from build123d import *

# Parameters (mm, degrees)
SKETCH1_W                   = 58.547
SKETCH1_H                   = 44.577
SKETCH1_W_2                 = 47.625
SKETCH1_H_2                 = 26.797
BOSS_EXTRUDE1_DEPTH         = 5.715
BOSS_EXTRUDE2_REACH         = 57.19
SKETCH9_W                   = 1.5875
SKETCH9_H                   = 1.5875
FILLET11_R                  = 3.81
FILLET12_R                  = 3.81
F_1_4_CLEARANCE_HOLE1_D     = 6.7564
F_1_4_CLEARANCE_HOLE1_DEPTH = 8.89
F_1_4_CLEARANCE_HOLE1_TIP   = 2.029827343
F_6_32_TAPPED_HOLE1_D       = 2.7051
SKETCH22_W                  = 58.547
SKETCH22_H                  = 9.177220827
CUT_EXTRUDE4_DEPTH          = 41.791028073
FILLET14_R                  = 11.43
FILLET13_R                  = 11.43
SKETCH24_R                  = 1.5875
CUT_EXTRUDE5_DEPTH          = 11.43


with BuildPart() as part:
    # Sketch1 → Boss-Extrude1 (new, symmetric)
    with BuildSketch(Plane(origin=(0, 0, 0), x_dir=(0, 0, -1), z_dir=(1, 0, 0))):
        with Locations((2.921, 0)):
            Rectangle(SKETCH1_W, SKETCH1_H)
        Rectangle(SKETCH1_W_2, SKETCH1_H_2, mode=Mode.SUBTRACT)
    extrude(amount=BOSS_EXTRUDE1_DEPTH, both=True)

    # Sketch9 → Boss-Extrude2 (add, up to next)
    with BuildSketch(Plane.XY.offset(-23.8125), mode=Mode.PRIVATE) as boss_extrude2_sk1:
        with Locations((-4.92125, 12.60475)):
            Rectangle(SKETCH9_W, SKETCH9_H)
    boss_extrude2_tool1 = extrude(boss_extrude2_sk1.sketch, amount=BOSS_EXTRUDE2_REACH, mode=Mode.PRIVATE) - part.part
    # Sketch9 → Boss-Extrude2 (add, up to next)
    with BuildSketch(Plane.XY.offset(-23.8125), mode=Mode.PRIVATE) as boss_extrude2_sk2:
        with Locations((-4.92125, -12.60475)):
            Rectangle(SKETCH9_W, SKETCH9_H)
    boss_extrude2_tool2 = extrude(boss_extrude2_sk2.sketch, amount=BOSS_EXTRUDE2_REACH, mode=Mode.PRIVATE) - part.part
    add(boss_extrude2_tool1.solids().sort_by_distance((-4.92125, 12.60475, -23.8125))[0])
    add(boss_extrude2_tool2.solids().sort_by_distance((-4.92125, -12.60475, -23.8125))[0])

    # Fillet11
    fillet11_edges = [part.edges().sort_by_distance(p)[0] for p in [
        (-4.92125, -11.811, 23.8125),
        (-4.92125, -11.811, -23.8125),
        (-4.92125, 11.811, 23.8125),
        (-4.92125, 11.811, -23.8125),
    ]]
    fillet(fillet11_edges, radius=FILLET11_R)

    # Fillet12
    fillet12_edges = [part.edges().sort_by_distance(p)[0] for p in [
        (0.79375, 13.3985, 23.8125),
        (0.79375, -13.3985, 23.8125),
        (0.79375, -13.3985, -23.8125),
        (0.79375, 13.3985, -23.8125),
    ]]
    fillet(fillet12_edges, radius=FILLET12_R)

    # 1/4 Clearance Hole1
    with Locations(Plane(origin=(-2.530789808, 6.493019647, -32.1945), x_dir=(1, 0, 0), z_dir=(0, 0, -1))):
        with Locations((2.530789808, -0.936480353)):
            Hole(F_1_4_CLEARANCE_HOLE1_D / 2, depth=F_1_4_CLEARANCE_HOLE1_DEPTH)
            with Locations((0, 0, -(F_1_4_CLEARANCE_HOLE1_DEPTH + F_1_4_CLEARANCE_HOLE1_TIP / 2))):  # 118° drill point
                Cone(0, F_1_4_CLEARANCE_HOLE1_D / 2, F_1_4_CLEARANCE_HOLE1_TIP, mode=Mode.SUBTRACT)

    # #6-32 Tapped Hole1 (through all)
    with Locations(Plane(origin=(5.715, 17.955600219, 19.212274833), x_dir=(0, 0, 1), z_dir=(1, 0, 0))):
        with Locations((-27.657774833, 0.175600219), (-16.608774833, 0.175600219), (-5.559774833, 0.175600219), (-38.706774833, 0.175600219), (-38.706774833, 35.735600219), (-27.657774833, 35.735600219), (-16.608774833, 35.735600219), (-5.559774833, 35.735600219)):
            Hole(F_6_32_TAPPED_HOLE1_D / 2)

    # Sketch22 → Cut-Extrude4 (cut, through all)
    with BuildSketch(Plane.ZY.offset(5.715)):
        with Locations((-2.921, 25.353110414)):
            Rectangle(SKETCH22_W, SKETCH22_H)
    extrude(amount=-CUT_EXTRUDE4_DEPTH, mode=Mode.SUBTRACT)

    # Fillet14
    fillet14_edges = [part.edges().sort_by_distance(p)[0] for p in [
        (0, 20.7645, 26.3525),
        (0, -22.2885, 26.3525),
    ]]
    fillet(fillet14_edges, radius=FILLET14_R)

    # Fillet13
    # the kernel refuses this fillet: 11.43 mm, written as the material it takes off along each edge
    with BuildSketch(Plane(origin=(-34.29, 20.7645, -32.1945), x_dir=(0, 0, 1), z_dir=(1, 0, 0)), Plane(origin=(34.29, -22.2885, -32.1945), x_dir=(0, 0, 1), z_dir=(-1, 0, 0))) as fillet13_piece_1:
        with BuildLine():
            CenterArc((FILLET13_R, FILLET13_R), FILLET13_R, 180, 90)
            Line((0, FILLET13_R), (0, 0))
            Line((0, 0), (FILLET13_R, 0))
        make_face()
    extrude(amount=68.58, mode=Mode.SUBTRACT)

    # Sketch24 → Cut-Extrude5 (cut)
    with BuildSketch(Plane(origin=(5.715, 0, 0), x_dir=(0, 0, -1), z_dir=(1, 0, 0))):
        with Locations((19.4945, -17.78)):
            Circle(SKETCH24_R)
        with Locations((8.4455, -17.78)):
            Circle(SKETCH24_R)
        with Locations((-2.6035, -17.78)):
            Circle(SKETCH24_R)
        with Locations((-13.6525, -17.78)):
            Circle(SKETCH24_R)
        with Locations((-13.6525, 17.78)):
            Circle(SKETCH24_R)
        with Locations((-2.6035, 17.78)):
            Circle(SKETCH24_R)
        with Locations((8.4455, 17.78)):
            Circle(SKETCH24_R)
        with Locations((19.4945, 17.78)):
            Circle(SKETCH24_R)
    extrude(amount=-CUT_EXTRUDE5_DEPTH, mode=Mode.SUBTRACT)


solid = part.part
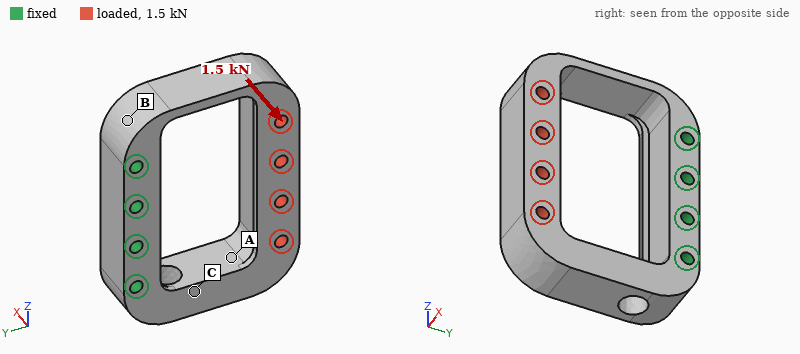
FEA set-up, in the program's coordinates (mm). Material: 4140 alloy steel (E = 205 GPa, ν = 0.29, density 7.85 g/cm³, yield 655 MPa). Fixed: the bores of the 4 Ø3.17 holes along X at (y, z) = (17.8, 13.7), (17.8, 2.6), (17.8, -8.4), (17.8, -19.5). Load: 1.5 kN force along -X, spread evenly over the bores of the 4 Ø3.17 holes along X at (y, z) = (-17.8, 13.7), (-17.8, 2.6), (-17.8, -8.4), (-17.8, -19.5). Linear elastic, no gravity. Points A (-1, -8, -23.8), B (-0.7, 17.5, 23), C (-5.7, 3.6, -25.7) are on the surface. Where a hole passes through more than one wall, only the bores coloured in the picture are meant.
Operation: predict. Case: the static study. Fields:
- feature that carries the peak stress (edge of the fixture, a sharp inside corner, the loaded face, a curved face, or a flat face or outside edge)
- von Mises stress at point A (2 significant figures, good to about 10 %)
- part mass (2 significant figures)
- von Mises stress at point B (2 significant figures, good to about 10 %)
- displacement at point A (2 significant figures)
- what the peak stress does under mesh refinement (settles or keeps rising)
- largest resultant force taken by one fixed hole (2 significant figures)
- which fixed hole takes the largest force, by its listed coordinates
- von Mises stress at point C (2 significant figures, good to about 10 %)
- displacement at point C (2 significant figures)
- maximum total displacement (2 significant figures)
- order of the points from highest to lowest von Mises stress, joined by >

edge of the fixture
46 MPa
97 g
200 MPa
0.10 mm
keeps rising
750 N
(17.8, -19.5)
120 MPa
0.053 mm
0.25 mm
B > C > A
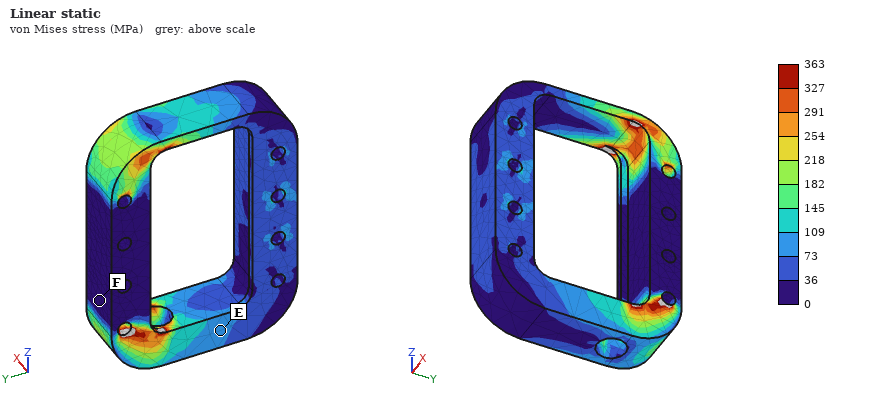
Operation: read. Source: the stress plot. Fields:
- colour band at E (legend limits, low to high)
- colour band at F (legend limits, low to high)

73 to 109 MPa
0 to 36 MPa
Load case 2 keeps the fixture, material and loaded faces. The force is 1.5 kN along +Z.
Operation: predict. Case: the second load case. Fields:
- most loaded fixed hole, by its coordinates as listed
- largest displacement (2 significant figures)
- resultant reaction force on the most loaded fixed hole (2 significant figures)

(17.8, -19.5)
0.13 mm
1.4 kN
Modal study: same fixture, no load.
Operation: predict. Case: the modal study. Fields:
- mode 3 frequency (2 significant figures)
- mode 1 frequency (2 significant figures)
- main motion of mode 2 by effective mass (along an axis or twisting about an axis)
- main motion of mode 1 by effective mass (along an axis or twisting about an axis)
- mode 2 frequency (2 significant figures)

4900 Hz
2100 Hz
along Z
along X
2500 Hz
